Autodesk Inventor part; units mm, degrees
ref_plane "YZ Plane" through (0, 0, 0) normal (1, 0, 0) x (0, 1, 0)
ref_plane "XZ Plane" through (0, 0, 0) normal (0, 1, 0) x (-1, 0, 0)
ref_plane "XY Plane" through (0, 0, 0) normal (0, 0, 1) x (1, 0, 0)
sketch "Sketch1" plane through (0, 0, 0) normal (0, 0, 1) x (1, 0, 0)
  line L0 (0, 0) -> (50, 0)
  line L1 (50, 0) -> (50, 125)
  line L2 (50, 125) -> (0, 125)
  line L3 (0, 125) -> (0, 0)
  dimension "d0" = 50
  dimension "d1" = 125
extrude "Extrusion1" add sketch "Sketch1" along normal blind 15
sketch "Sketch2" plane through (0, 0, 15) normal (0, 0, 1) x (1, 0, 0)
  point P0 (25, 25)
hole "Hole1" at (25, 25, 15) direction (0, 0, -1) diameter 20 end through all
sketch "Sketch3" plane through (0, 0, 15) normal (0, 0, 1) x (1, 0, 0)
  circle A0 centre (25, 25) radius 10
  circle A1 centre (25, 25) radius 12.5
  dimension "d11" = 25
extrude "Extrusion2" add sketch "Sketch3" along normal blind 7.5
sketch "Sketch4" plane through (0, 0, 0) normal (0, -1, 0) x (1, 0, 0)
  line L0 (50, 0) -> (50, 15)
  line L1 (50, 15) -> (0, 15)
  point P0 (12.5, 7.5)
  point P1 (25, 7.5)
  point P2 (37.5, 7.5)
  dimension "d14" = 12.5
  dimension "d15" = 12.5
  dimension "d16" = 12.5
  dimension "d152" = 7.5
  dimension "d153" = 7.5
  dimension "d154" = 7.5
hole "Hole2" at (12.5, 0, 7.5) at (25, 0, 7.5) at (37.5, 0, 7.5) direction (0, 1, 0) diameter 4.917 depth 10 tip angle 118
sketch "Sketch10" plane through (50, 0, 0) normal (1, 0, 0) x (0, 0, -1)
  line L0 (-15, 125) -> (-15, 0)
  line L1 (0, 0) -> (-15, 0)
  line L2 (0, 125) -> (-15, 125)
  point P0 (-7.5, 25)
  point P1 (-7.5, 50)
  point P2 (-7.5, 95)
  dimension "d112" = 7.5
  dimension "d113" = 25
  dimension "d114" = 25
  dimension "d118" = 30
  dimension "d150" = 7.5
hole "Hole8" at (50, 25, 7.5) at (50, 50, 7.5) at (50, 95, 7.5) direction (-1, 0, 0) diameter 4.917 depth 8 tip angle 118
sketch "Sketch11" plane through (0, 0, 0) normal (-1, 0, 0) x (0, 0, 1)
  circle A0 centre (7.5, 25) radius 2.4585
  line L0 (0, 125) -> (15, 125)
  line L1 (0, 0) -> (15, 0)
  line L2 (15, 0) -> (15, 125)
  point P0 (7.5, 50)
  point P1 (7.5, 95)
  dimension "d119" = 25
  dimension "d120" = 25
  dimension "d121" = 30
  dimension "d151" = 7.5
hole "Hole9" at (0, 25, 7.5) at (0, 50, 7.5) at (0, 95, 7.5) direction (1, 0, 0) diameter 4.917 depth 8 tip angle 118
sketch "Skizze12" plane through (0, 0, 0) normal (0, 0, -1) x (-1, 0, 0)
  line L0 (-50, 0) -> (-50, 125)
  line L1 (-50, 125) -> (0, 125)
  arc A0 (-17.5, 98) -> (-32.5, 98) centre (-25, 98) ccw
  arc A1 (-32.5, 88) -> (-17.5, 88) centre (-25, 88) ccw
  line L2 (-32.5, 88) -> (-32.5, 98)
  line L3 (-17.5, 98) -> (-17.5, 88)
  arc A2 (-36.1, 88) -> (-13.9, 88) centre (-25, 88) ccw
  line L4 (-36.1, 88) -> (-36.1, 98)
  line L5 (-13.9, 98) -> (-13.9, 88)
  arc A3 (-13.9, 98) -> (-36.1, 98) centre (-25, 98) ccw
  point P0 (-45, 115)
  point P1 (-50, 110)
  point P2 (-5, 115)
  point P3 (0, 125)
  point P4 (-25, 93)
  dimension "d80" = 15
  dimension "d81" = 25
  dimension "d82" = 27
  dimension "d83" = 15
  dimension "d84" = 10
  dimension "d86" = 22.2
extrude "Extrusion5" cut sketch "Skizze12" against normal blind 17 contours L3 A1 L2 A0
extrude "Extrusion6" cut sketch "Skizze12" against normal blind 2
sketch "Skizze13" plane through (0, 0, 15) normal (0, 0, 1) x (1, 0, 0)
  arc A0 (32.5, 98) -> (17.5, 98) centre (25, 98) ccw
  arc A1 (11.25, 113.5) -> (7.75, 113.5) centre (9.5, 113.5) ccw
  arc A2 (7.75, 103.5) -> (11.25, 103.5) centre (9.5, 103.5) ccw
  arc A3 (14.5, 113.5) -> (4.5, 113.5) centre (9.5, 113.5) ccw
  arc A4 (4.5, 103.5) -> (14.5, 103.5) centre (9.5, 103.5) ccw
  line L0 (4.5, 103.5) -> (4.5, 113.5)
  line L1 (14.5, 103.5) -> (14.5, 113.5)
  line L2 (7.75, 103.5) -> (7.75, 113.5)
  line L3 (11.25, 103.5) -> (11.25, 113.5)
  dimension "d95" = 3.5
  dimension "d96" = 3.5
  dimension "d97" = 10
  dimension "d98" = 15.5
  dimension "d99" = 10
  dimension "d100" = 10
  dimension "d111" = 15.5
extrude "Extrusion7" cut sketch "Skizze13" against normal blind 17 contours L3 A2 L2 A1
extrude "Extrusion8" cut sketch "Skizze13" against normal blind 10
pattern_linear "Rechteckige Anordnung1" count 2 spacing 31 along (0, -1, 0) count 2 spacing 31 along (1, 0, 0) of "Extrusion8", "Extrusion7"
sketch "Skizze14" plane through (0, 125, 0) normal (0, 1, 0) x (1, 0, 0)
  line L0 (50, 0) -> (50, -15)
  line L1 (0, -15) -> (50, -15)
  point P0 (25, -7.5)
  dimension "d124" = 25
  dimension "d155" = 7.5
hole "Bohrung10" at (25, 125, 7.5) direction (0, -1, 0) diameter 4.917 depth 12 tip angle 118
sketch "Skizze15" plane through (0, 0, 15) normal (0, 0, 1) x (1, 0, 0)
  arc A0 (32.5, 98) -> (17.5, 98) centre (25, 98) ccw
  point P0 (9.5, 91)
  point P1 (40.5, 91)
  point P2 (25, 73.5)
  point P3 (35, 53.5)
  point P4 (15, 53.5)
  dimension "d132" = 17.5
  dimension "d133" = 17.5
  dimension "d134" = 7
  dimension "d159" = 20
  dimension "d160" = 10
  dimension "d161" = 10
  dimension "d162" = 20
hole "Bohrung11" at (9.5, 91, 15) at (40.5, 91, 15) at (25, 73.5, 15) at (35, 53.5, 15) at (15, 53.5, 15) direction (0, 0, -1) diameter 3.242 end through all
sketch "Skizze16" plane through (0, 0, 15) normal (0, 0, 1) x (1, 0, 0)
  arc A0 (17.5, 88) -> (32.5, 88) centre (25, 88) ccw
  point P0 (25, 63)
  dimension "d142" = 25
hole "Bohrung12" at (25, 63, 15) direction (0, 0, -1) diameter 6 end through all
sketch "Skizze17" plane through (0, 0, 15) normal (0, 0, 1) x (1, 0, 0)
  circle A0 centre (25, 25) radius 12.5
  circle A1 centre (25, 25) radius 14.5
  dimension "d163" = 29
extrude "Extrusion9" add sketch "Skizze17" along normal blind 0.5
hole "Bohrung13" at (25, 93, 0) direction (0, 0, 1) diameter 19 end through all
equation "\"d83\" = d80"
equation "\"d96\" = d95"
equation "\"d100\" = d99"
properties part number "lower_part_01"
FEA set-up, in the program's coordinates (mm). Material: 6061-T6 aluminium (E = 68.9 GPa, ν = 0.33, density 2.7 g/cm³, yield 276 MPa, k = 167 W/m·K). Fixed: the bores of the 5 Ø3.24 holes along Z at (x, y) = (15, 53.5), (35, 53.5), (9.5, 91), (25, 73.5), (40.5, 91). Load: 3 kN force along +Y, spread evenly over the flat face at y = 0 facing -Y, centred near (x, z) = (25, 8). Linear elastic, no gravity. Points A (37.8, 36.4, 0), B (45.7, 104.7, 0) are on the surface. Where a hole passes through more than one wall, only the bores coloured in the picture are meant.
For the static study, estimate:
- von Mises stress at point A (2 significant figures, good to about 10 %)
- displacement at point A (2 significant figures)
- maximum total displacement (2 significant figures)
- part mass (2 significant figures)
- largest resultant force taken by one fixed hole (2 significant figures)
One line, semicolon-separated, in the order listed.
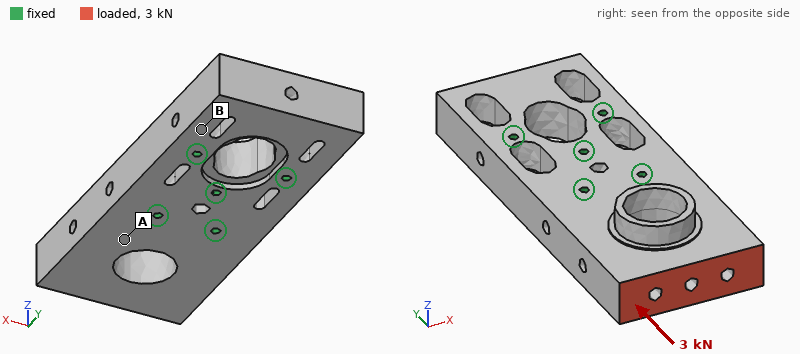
8.0 MPa; 1.9 µm; 6.7 µm; 200 g; 1.2 kN
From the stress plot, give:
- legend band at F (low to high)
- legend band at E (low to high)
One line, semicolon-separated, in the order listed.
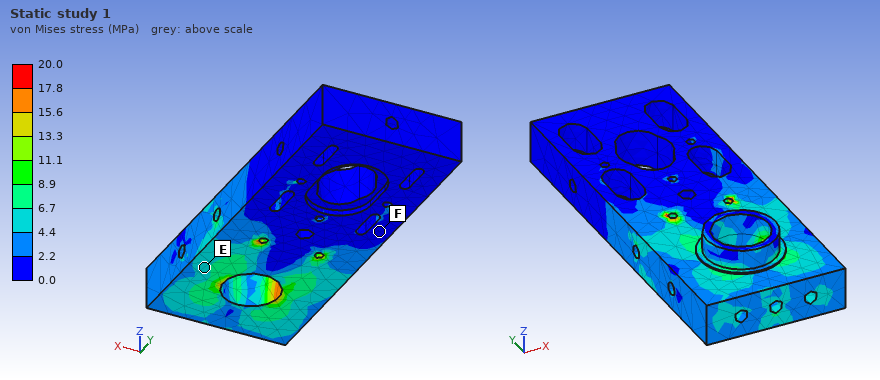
0.0 to 2.2 MPa; 4.4 to 6.7 MPa
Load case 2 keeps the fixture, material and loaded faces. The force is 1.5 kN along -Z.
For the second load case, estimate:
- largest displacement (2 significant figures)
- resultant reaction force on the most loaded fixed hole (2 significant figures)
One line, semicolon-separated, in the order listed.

0.12 mm; 1.3 kN
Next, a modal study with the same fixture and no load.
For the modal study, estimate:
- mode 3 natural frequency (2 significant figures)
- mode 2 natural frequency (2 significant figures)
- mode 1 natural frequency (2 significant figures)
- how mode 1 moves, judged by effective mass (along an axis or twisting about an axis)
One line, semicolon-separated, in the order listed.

6700 Hz; 6500 Hz; 3600 Hz; along Z
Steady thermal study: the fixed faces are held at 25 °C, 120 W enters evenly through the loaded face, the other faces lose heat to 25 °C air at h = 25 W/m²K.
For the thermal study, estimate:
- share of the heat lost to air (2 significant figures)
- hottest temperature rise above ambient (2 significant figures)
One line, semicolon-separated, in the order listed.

7.0 %; 66 K
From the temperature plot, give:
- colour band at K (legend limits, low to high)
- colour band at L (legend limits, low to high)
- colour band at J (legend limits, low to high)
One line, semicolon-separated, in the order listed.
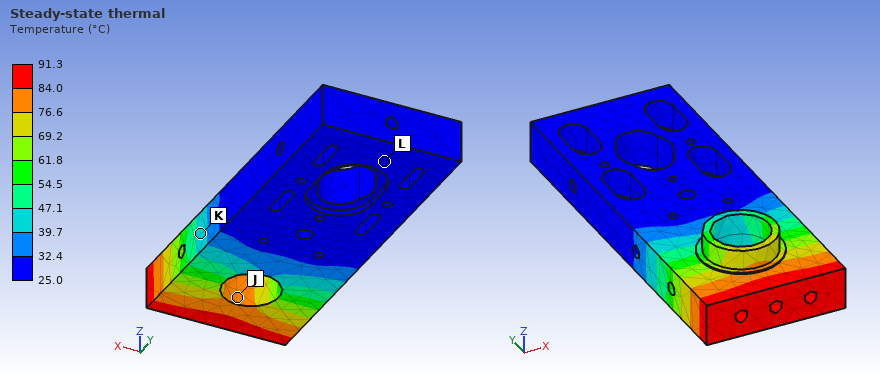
39.7 to 47.1 °C; 25.0 to 32.4 °C; 76.6 to 84.0 °C
